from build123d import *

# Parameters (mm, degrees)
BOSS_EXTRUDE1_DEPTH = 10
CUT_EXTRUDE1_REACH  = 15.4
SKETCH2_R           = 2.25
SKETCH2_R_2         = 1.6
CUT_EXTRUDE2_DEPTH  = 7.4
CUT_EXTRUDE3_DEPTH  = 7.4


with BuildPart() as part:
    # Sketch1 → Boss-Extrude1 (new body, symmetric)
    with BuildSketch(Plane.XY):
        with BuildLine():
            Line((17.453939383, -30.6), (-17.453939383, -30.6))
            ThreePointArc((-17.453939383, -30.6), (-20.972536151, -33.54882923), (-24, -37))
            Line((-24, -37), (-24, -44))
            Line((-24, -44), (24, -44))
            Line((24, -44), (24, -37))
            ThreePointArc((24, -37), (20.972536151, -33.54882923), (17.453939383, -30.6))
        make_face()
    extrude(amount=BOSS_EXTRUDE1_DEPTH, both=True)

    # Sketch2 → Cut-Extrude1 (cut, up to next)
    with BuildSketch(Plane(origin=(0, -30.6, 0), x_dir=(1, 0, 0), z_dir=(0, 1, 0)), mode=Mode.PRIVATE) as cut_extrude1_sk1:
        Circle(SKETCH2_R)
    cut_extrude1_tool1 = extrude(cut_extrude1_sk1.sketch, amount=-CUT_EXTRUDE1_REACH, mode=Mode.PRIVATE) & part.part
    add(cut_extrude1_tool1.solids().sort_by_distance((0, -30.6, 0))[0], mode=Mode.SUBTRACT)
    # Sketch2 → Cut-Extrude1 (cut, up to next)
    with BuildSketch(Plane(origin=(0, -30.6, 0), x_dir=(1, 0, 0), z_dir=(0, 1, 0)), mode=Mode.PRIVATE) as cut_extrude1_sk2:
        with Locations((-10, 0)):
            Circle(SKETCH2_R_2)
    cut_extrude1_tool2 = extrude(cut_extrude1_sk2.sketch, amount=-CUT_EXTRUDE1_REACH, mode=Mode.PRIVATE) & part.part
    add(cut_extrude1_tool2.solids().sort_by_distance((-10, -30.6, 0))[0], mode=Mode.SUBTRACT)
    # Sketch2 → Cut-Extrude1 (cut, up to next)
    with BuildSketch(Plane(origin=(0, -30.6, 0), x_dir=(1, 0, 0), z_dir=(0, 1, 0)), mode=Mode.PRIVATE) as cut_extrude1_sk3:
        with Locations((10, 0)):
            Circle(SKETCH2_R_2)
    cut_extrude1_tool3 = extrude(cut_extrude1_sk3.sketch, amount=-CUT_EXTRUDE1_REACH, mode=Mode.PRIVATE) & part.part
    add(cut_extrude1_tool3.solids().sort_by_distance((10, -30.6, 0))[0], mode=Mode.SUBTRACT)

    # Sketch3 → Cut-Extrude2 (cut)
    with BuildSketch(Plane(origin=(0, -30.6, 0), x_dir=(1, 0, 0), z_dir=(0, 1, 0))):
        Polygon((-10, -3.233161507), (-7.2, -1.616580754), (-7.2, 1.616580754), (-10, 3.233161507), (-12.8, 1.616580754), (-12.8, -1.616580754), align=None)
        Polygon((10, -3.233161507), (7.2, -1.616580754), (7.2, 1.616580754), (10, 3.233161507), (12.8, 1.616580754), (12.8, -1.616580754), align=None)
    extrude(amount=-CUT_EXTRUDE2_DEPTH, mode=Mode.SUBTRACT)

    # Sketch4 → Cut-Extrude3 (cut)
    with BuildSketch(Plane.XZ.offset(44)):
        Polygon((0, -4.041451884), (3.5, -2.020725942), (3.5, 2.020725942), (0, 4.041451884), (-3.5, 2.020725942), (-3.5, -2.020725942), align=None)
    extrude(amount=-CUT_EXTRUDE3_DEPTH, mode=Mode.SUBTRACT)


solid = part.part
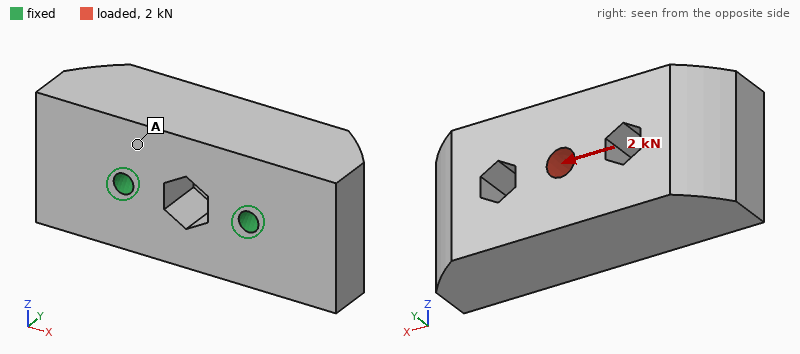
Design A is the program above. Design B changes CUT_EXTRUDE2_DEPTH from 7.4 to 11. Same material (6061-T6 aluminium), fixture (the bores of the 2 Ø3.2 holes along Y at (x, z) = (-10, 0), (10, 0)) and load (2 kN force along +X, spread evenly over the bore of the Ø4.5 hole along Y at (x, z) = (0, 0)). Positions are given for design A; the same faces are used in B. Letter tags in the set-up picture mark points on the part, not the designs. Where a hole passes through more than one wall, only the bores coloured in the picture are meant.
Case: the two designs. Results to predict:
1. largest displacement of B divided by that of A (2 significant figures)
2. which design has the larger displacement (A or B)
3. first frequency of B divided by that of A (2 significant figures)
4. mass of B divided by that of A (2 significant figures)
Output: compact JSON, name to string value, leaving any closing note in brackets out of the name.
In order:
{"largest displacement of B divided by that of A": "2.3", "which design has the larger displacement": "B", "first frequency of B divided by that of A": "0.38", "mass of B divided by that of A": "0.99"}
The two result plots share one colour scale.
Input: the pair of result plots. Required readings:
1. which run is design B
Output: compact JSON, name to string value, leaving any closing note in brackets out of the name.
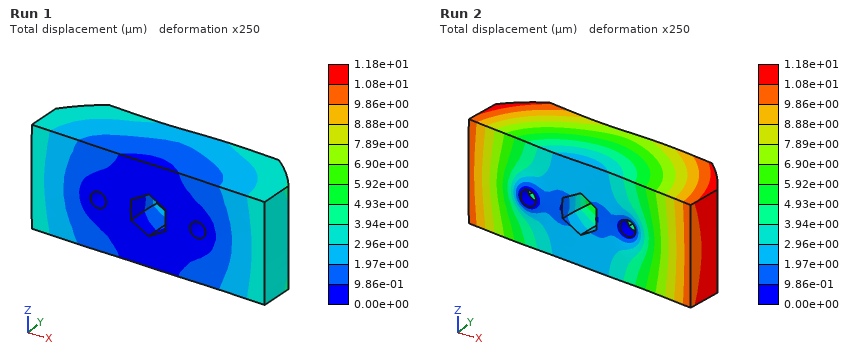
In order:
{"which run is design B": "Run 2"}
